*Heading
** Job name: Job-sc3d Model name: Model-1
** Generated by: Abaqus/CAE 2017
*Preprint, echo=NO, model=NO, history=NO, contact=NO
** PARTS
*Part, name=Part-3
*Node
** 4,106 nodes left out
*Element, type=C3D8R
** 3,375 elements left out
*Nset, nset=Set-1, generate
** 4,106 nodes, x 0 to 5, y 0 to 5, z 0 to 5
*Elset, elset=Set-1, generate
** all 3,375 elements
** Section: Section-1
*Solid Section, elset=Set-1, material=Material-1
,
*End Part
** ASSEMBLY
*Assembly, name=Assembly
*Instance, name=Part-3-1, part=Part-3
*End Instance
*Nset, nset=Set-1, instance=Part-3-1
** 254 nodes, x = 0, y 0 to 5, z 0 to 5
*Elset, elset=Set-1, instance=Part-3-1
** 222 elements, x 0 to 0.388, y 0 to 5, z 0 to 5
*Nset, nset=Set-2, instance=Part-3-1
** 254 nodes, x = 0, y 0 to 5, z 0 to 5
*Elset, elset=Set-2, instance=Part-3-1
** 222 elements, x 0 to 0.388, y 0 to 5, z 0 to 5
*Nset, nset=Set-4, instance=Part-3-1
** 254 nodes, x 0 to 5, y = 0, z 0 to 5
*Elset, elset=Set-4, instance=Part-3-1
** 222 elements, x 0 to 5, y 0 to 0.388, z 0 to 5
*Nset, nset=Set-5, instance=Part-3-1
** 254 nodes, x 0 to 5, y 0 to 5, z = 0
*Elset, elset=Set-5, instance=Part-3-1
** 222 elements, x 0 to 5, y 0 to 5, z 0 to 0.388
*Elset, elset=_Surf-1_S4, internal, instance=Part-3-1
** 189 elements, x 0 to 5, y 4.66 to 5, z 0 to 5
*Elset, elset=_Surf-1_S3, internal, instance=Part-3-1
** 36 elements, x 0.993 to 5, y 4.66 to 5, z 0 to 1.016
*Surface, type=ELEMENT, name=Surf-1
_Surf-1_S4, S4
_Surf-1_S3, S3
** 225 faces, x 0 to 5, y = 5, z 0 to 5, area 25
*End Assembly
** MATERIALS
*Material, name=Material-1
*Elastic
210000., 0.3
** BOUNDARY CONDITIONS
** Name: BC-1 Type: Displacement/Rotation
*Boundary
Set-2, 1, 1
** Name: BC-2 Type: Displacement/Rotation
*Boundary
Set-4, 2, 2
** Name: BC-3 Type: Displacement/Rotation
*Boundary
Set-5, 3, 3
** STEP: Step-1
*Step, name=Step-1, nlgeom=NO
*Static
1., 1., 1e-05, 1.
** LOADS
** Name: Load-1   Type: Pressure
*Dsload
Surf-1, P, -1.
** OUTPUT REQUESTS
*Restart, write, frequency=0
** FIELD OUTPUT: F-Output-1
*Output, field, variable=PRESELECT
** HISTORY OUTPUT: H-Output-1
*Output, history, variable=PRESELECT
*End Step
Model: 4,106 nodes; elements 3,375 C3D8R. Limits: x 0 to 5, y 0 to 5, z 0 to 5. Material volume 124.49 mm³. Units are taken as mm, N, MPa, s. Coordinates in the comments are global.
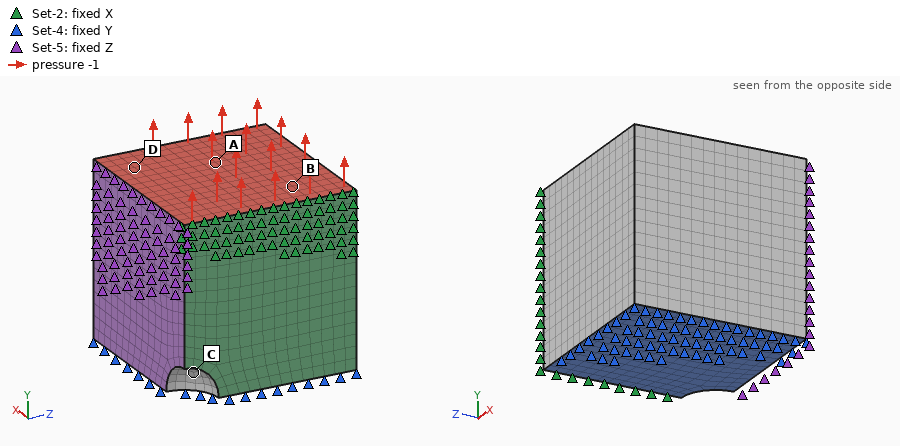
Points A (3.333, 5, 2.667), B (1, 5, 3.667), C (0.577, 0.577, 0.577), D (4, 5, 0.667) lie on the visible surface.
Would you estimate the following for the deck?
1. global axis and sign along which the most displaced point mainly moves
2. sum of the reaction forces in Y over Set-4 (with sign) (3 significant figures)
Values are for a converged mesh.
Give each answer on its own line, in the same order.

+Y
-25.0 N
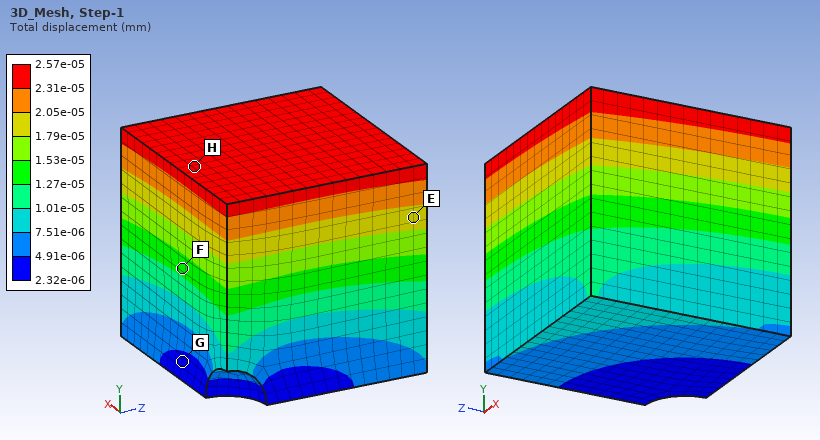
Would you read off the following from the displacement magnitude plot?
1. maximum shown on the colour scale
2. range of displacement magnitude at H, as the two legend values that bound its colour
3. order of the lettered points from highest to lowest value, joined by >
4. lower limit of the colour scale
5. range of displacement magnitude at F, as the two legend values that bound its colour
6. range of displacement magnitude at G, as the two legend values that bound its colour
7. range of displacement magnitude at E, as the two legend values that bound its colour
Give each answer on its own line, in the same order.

2.57e-05 mm
2.31e-05 to 2.57e-05 mm
H > E > F > G
2.32e-06 mm
1.27e-05 to 1.53e-05 mm
2.32e-06 to 4.91e-06 mm
1.79e-05 to 2.05e-05 mm
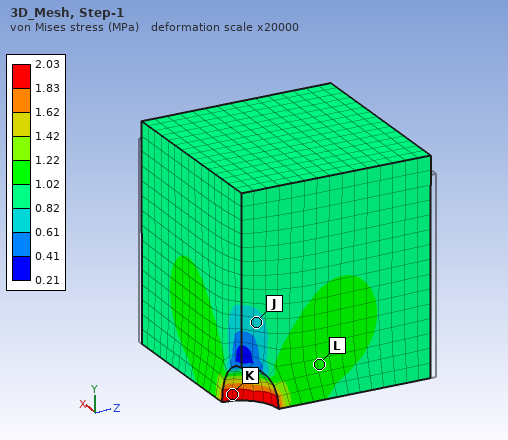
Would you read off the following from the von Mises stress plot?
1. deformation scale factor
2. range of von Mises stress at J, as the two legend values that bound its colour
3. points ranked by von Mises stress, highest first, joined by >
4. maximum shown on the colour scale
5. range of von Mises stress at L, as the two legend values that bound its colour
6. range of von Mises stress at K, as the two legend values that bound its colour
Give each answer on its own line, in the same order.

20000
0.61 to 0.82 MPa
K > L > J
2.03 MPa
1.02 to 1.22 MPa
1.83 to 2.03 MPa
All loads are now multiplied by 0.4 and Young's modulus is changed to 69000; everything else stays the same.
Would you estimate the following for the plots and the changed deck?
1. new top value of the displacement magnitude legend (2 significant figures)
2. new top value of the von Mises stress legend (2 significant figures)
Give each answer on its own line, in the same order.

3.1e-05 mm
0.81 MPa
